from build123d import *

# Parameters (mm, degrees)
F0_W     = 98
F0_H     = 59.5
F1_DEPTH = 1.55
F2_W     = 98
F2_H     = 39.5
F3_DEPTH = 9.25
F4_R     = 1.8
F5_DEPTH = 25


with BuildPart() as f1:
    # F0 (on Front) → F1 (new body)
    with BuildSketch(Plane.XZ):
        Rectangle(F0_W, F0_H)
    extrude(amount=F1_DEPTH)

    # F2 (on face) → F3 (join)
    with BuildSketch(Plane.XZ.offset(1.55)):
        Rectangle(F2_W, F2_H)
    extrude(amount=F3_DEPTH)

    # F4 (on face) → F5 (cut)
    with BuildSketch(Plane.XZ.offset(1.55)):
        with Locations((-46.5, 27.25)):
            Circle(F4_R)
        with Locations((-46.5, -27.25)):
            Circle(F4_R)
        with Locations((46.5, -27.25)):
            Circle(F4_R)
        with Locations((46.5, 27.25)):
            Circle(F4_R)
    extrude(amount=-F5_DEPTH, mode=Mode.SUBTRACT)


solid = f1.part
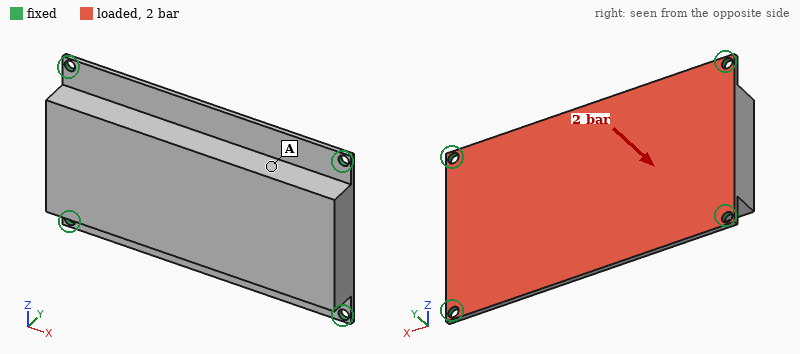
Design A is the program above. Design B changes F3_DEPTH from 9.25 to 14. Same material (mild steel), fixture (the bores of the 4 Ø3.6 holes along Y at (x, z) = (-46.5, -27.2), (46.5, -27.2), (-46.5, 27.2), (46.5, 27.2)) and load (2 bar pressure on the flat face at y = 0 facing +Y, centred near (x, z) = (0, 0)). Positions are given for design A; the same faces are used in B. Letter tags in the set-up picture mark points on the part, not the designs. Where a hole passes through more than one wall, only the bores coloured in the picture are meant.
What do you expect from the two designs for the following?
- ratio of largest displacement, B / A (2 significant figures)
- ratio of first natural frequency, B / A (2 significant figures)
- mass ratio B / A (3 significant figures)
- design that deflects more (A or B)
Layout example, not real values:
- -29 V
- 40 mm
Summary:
- 0.79
- 0.92
- 1.41
- A
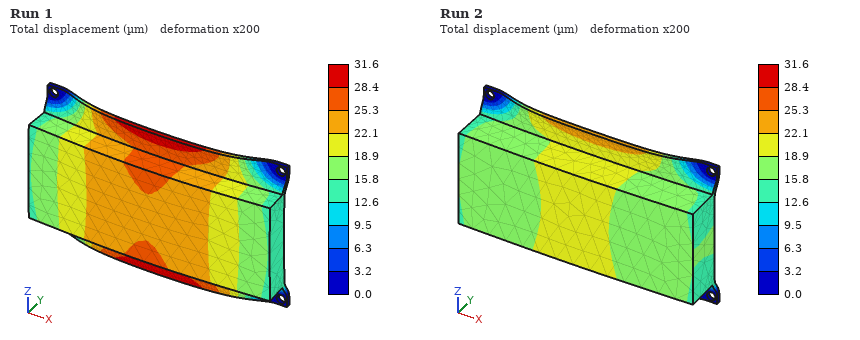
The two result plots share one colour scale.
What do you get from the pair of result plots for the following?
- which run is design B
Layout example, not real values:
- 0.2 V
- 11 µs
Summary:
- Run 2
